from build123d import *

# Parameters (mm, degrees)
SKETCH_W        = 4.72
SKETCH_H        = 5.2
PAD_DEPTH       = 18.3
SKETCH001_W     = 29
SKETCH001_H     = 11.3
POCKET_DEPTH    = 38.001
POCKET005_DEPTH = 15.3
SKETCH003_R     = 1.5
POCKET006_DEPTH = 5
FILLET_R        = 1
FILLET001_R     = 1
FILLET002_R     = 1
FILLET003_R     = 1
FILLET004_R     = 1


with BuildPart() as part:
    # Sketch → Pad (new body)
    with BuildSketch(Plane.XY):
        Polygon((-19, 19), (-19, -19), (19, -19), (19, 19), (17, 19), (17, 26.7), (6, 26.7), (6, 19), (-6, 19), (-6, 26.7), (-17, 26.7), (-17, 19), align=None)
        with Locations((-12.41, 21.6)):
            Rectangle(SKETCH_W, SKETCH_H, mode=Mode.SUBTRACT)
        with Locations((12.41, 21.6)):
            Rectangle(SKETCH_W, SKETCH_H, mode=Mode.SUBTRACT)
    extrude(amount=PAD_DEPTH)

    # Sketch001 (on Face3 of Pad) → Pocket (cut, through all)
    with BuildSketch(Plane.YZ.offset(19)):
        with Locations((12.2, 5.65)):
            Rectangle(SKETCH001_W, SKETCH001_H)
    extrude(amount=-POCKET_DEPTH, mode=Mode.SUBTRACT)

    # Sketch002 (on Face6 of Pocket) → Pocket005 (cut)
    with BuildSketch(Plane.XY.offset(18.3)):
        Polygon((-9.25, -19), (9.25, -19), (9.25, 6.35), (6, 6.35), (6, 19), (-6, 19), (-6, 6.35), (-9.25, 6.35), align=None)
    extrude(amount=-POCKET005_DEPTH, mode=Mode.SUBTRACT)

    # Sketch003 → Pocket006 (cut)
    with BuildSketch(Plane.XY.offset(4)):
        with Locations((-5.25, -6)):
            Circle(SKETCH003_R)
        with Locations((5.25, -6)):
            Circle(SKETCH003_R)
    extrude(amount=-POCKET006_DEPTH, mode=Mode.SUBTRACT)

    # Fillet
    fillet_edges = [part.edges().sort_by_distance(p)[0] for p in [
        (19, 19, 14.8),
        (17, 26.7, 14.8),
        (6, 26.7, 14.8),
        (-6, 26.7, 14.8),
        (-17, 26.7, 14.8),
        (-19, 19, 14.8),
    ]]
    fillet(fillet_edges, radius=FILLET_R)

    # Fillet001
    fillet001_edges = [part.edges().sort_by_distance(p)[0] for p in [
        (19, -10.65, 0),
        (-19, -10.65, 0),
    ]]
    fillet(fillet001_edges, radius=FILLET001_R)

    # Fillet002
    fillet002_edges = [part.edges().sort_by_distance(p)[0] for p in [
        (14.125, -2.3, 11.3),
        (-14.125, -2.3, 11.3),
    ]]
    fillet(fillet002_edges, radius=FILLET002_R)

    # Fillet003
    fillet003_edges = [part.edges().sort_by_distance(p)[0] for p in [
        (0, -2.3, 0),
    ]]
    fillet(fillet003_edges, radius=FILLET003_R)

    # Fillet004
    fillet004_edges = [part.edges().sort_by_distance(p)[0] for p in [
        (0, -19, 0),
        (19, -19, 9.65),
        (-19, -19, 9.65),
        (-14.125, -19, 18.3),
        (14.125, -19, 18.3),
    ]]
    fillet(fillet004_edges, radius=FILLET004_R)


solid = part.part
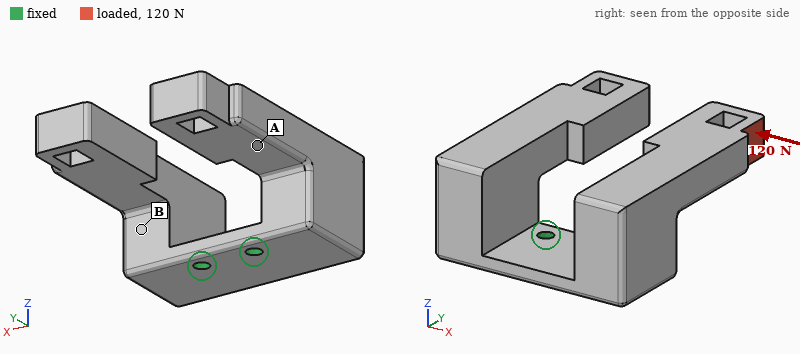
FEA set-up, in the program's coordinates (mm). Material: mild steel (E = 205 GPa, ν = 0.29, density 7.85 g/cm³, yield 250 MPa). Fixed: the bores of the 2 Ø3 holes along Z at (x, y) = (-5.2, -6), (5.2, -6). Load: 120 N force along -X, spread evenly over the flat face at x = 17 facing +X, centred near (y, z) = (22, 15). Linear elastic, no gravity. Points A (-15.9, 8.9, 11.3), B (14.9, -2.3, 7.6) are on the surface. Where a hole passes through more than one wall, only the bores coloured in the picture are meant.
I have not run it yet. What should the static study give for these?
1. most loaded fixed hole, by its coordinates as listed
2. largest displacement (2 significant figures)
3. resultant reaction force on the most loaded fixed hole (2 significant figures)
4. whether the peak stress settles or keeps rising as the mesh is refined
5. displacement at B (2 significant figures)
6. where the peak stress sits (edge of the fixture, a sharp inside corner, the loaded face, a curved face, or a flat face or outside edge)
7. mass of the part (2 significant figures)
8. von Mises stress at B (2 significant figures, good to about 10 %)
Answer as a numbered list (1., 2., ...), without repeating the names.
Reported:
1. (5.2, -6)
2. 48 µm
3. 340 N
4. keeps rising
5. 13 µm
6. edge of the fixture
7. 87 g
8. 21 MPa
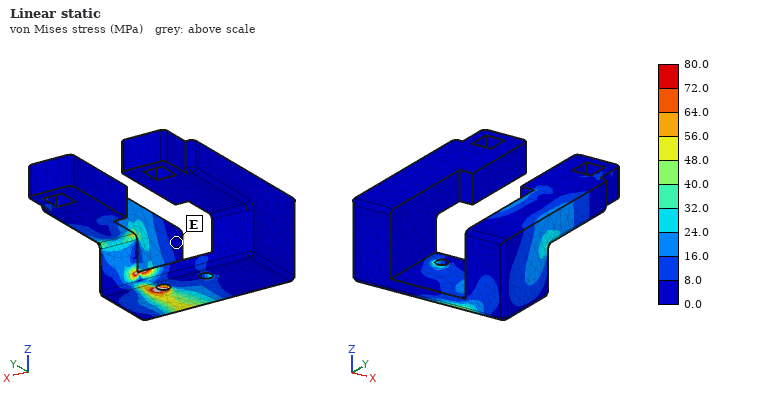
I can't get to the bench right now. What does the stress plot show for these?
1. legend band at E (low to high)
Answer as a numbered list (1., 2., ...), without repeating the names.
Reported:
1. 0.0 to 8.0 MPa
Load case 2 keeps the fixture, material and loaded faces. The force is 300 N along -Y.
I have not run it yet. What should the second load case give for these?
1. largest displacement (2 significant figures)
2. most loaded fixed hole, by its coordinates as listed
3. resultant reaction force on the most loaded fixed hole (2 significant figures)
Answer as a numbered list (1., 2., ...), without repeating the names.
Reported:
1. 67 µm
2. (5.2, -6)
3. 530 N
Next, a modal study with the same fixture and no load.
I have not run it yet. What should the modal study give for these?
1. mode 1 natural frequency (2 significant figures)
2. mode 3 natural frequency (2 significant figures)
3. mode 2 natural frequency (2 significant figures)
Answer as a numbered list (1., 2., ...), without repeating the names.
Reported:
1. 1900 Hz
2. 2100 Hz
3. 2000 Hz
